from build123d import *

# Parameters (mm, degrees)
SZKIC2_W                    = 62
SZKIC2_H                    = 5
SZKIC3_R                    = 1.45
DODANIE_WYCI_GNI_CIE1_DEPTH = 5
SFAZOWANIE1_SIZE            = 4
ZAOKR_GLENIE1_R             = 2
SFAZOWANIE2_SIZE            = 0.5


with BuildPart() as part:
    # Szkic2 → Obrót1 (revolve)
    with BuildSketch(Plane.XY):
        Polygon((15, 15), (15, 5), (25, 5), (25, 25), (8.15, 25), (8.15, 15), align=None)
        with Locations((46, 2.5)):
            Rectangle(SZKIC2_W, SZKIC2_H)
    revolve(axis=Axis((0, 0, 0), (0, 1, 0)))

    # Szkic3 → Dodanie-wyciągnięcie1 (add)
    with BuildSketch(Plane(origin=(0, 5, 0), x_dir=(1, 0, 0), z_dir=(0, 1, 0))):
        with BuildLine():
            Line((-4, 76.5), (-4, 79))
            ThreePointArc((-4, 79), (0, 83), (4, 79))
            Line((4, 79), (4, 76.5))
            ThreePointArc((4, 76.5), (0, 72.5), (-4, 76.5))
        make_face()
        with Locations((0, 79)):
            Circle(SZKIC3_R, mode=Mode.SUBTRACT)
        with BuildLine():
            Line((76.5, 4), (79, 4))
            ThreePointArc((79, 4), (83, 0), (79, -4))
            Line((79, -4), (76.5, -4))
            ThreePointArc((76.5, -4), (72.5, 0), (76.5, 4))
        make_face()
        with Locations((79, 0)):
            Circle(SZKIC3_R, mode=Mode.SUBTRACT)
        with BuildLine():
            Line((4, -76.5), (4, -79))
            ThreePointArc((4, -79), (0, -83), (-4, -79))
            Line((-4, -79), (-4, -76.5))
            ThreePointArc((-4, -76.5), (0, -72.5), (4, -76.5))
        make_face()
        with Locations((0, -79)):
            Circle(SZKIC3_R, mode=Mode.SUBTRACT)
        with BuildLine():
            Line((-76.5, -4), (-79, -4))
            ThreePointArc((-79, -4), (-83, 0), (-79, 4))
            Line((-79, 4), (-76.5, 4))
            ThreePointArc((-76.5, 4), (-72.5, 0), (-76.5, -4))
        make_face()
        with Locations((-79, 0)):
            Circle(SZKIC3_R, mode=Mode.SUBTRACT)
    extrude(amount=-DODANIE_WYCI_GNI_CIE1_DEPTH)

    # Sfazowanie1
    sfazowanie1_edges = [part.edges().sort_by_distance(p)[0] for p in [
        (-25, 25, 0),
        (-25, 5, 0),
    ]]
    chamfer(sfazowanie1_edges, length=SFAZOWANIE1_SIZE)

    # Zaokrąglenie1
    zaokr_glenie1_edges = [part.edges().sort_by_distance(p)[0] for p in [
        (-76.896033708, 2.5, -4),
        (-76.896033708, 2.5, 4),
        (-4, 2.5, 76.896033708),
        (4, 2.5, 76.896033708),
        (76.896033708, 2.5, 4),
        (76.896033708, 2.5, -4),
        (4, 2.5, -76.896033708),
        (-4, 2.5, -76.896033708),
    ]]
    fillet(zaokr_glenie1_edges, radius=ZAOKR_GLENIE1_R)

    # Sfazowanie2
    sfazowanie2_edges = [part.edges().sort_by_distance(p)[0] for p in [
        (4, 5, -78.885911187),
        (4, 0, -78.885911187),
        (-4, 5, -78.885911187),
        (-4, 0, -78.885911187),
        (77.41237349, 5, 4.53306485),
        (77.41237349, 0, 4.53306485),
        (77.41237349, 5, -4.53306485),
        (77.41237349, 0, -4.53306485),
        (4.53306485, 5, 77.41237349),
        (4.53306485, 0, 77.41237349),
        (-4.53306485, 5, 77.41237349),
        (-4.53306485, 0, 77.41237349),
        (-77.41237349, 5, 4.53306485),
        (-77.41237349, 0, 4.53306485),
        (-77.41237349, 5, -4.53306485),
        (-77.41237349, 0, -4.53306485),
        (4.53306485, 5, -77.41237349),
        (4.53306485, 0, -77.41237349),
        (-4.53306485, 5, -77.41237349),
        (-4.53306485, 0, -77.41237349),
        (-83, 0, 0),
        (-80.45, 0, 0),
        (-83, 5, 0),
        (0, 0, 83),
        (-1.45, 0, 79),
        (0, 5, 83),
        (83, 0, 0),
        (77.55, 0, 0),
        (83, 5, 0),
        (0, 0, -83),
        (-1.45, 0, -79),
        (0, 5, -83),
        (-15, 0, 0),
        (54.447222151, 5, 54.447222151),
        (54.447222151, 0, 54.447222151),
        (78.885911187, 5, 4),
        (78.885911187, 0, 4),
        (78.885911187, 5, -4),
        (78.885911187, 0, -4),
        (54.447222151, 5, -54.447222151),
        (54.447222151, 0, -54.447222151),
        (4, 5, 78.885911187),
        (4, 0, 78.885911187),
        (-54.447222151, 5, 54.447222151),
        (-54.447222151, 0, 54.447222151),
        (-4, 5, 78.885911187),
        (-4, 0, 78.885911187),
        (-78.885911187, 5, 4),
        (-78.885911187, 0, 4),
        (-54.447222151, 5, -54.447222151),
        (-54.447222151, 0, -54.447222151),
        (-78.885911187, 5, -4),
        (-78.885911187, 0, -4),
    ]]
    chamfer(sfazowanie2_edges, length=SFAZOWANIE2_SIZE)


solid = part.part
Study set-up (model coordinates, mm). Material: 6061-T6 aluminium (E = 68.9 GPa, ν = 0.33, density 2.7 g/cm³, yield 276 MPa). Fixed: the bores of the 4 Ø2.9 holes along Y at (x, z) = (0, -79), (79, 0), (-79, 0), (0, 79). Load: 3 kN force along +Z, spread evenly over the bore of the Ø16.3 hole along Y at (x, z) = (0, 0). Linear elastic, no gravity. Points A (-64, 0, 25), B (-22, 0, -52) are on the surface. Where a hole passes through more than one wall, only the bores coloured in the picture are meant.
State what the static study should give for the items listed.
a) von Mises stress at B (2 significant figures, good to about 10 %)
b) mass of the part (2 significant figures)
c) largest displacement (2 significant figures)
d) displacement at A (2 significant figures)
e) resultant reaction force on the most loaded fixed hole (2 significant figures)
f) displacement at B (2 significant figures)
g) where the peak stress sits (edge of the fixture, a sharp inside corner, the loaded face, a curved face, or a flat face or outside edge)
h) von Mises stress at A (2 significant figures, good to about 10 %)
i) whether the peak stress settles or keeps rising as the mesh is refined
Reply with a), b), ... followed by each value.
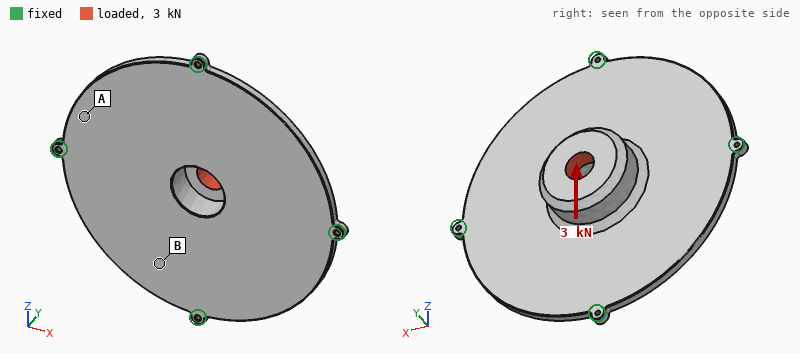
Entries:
a) 15 MPa
b) 330 g
c) 97 µm
d) 42 µm
e) 1.1 kN
f) 68 µm
g) edge of the fixture
h) 6.6 MPa
i) keeps rising
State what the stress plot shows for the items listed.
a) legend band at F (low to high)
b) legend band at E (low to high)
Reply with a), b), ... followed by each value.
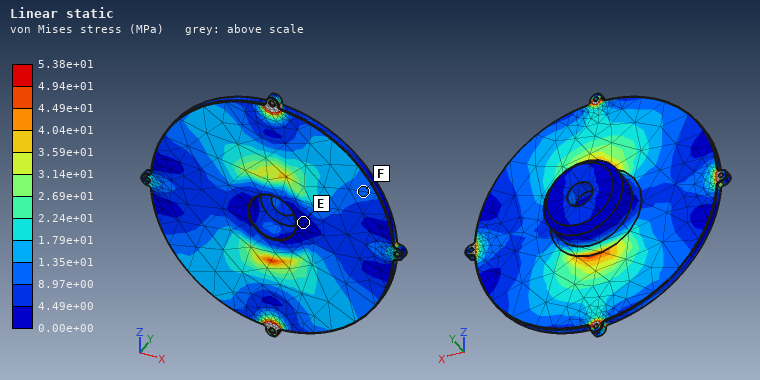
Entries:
a) 8.97e+00 to 1.35e+01 MPa
b) 0.00e+00 to 4.49e+00 MPa
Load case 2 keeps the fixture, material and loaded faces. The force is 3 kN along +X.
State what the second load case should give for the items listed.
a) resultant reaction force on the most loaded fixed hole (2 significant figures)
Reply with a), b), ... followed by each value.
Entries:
a) 1.1 kN
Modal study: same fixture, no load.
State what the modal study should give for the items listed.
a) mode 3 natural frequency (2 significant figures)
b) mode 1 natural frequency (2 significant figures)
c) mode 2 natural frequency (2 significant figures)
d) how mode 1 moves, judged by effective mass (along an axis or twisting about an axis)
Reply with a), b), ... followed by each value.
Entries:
a) 1700 Hz
b) 1000 Hz
c) 1700 Hz
d) along Y
